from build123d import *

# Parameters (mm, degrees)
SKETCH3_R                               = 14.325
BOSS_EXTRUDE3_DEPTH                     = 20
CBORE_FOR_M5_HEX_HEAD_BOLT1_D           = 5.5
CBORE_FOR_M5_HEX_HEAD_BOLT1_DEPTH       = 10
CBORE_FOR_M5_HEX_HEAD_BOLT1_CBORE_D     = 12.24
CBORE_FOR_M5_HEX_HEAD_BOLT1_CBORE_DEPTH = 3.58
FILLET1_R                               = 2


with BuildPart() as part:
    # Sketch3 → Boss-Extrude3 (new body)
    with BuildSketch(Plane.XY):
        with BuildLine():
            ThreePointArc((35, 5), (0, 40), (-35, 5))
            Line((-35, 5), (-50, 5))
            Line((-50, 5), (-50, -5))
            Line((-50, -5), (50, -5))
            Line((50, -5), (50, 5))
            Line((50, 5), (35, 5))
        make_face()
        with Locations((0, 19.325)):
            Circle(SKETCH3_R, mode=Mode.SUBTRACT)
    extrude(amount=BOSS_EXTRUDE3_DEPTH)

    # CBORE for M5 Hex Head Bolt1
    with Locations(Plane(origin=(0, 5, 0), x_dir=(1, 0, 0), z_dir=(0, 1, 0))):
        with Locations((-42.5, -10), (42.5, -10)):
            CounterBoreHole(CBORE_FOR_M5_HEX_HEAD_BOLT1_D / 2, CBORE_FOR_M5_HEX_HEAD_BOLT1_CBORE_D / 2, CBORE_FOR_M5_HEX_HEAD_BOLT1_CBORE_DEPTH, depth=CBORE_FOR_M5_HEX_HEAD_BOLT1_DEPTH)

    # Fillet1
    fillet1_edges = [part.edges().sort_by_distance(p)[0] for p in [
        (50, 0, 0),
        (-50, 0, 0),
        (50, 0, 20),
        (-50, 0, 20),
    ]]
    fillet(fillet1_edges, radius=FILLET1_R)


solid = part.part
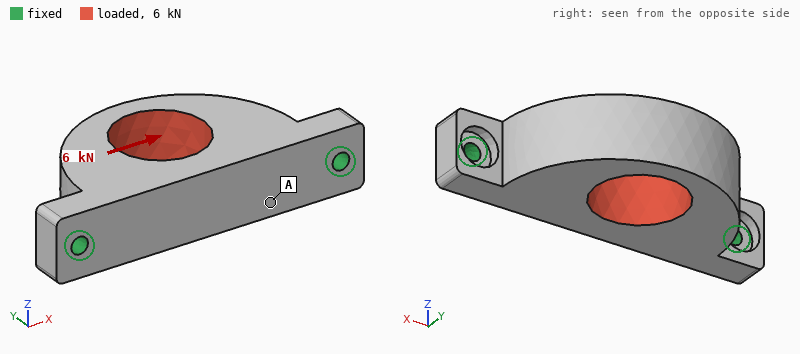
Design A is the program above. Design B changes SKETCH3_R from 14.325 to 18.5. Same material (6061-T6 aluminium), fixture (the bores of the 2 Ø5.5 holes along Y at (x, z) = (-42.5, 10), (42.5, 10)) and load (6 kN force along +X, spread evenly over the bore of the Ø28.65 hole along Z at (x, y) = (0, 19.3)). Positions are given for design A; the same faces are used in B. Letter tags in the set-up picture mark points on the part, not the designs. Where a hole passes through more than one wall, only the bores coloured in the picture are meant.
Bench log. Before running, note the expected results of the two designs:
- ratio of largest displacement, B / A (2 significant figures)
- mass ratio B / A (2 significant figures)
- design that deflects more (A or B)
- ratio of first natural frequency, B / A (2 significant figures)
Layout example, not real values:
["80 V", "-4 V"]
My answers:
["2.9", "0.81", "B", "1.2"]
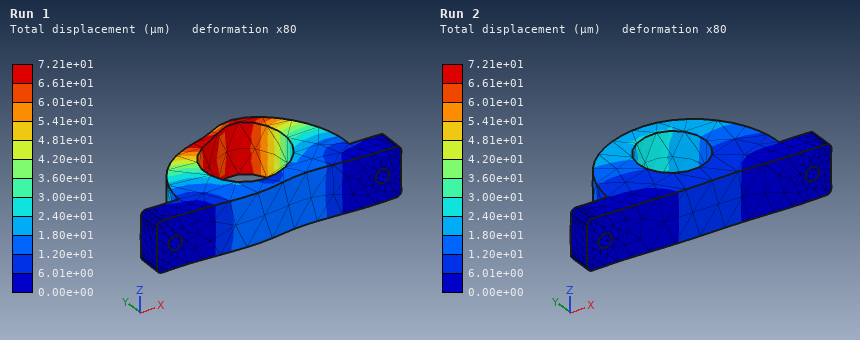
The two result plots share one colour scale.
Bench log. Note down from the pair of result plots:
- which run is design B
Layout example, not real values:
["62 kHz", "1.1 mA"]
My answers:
["Run 1"]
